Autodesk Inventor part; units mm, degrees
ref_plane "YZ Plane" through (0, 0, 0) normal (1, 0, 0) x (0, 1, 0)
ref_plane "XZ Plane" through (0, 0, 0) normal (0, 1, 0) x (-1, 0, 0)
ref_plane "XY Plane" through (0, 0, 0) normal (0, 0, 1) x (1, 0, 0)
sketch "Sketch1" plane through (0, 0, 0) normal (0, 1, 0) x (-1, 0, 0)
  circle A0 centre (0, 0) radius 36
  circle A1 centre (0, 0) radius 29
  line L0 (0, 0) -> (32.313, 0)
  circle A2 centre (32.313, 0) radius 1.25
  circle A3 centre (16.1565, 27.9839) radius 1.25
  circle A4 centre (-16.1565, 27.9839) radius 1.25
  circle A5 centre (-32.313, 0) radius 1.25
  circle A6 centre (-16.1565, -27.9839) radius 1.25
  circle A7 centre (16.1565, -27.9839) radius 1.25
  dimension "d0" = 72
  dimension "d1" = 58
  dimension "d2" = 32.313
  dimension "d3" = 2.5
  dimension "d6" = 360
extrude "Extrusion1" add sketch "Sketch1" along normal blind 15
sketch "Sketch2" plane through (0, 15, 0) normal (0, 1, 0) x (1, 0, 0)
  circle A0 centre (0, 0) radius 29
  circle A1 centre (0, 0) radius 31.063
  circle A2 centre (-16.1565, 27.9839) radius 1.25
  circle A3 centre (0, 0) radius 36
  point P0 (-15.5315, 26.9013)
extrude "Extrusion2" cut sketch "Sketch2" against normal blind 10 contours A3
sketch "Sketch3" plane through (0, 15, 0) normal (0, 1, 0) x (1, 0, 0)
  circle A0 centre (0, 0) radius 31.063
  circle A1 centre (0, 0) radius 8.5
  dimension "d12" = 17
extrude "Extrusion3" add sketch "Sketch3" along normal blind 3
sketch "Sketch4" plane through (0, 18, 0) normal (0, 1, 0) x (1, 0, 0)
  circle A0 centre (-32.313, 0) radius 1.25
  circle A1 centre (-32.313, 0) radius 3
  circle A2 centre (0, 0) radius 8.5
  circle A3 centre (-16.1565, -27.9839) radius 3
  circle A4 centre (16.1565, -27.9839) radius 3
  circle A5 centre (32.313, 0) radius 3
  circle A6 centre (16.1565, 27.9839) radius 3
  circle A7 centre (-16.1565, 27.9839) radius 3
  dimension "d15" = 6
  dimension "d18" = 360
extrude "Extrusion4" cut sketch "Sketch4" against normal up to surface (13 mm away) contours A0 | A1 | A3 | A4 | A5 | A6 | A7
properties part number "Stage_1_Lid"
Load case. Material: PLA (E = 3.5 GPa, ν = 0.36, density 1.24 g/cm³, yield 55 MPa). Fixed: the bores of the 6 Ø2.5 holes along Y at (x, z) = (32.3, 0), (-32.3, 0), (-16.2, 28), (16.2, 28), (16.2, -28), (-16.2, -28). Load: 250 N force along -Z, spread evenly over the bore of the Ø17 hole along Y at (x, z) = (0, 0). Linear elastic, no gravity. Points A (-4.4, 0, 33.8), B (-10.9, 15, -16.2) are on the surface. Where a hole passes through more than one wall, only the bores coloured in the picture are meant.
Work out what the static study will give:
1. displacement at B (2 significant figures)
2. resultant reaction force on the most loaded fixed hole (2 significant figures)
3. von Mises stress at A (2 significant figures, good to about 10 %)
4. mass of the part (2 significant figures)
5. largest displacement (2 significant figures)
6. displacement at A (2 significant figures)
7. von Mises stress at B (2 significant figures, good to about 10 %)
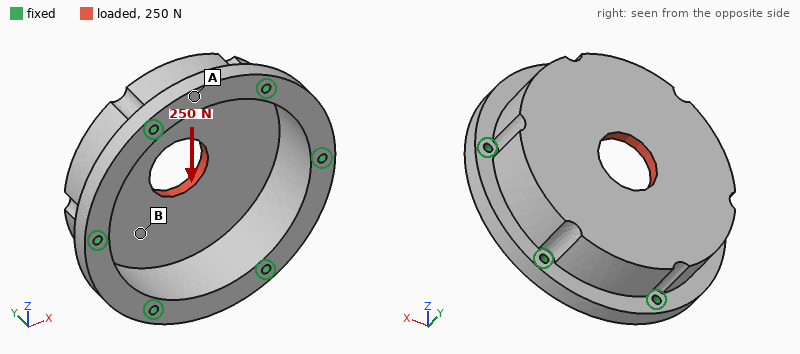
34 µm
66 N
0.60 MPa
23 g
41 µm
8.1 µm
1.6 MPa
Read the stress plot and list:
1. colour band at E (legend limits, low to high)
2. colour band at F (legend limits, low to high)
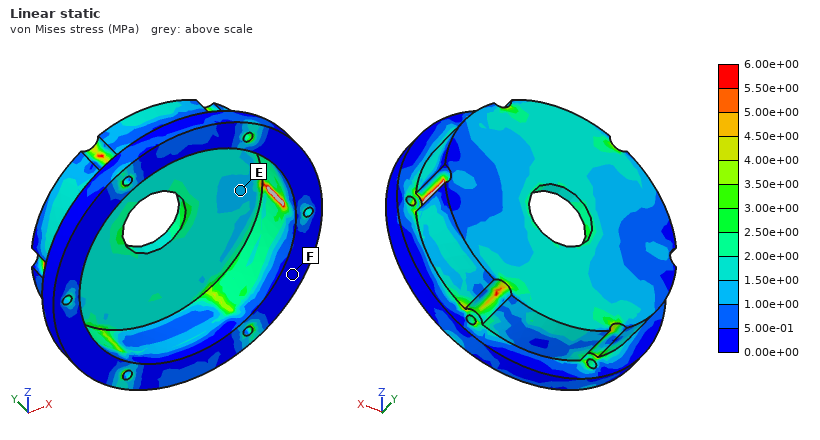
1.00e+00 to 1.50e+00 MPa
0.00e+00 to 5.00e-01 MPa
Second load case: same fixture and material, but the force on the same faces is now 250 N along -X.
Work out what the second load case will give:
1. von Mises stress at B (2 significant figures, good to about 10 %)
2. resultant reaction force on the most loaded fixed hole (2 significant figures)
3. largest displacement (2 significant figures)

1.6 MPa
60 N
41 µm
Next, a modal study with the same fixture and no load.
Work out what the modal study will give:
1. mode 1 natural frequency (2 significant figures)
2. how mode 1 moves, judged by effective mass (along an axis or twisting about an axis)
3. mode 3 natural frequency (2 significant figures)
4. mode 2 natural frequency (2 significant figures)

2100 Hz
along Y
3900 Hz
3900 Hz
